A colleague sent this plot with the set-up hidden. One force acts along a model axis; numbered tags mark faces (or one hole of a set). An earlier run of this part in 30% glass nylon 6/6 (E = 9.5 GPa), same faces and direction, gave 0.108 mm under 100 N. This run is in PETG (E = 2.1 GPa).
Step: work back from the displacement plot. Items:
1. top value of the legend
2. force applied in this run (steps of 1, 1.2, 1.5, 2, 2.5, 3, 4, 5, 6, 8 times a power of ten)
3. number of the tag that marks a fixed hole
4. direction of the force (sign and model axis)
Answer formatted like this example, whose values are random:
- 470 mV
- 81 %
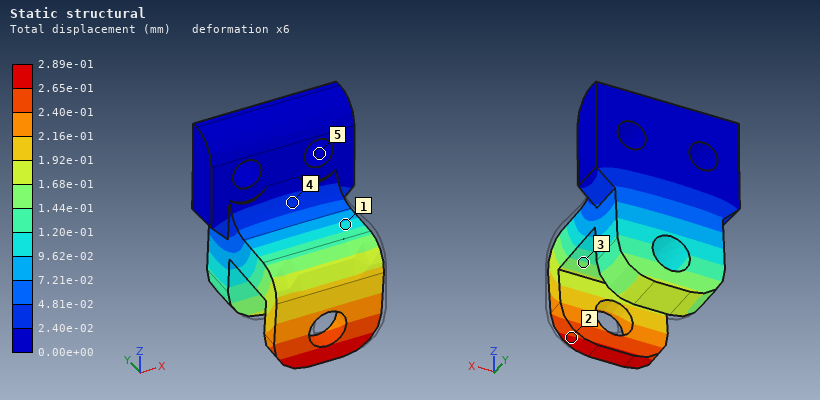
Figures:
- 2.89e-01 mm
- 60 N
- 5
- -Z
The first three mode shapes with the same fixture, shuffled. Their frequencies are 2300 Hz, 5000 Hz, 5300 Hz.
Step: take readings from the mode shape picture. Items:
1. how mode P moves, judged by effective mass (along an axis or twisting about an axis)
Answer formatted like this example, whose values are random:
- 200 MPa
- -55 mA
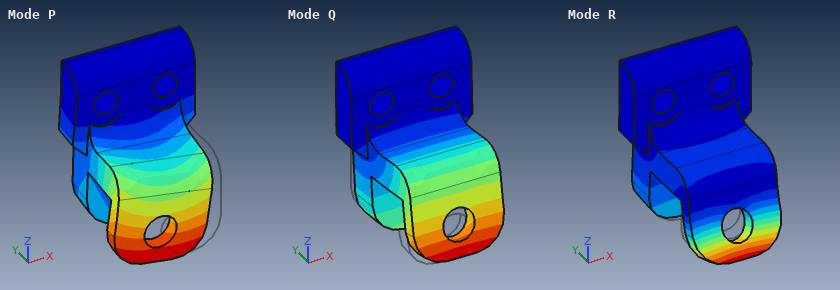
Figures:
- along X
